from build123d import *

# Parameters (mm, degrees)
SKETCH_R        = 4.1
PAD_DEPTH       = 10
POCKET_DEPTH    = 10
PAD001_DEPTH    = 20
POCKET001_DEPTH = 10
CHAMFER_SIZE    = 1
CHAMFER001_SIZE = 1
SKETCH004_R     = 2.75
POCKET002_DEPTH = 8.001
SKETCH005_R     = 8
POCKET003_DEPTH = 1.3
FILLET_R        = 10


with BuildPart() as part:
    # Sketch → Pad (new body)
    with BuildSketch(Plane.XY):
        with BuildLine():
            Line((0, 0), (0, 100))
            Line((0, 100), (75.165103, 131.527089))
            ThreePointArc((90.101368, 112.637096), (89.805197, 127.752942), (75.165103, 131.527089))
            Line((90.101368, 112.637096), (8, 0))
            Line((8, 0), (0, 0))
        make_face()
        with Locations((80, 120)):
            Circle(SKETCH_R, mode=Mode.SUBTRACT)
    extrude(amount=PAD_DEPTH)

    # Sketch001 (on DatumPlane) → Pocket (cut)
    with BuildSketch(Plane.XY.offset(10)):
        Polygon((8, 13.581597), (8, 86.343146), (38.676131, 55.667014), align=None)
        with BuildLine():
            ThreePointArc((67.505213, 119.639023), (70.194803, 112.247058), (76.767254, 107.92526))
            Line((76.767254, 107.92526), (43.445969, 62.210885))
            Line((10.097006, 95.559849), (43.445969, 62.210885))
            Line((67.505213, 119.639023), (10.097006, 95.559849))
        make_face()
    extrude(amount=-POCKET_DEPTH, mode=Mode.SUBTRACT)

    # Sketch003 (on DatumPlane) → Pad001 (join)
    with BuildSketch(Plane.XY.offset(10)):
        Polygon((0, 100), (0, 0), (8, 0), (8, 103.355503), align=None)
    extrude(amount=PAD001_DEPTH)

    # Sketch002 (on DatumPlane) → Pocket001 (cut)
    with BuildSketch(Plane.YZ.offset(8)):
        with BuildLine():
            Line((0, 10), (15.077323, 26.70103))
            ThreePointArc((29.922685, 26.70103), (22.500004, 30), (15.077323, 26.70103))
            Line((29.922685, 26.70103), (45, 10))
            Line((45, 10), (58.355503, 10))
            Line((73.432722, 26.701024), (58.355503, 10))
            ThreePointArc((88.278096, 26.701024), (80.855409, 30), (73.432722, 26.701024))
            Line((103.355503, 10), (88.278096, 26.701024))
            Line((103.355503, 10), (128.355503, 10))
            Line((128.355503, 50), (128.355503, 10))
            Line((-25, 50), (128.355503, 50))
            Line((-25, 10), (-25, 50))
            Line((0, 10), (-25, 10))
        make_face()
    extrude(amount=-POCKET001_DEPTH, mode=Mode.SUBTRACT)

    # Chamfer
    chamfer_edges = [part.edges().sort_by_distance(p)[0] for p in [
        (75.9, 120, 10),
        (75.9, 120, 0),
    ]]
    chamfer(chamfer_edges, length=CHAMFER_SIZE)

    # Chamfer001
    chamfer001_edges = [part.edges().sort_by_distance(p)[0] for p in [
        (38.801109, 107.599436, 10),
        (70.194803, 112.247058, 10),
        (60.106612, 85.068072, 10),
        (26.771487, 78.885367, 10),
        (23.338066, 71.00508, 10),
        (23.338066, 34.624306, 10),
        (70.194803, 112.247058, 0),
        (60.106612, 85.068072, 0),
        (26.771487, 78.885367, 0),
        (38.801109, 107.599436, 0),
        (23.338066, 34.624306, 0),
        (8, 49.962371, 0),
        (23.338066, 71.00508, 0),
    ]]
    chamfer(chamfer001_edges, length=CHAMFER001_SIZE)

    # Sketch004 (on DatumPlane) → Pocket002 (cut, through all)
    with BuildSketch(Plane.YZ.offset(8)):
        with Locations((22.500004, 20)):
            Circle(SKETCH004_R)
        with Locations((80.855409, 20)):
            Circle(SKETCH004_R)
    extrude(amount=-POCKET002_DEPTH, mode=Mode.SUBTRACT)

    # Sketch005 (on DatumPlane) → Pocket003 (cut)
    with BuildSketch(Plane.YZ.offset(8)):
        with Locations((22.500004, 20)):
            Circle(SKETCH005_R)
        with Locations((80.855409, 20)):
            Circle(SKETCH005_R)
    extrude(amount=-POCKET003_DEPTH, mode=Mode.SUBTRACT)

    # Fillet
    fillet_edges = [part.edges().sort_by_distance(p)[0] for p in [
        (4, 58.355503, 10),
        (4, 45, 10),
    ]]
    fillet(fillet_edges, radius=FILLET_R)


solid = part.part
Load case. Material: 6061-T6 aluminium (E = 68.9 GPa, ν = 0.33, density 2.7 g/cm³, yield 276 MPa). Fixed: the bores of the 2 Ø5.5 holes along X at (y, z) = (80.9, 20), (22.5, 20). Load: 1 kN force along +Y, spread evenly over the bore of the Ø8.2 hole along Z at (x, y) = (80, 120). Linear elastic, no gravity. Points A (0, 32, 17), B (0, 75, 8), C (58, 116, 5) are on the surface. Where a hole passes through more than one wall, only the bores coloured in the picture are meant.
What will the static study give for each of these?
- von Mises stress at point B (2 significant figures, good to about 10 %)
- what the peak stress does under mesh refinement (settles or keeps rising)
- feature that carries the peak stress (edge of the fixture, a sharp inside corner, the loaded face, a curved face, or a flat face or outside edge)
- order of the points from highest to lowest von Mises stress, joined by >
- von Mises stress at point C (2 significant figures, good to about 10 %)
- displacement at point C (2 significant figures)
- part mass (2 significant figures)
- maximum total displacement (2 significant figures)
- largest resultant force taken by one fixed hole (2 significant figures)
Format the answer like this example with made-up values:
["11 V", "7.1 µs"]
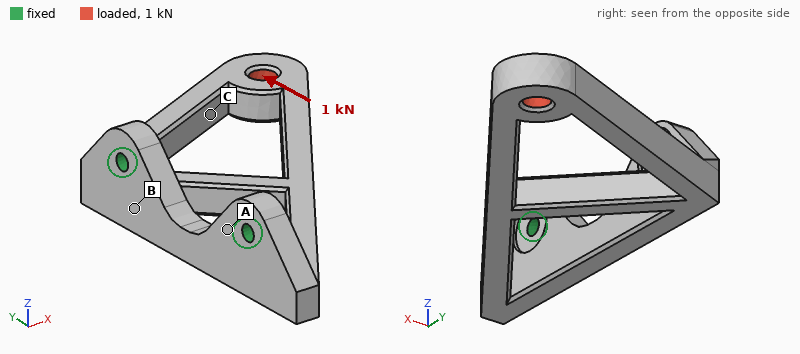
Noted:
["27 MPa", "keeps rising", "edge of the fixture", "C > B > A", "43 MPa", "0.24 mm", "110 g", "0.27 mm", "1.2 kN"]
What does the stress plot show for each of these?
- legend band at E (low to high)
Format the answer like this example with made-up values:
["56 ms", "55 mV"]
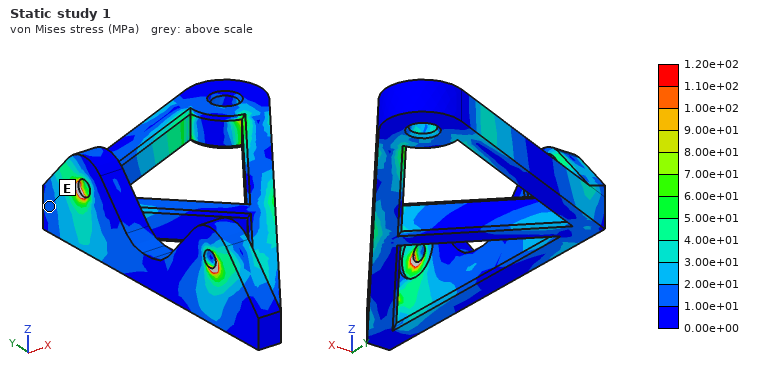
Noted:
["1.00e+01 to 2.00e+01 MPa"]
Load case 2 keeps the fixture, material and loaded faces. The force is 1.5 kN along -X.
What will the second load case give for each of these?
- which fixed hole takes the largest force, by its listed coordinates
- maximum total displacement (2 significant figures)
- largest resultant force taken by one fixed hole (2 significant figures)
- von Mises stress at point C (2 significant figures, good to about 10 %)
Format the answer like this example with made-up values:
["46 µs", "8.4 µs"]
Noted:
["(80.9, 20)", "0.48 mm", "2.1 kN", "66 MPa"]
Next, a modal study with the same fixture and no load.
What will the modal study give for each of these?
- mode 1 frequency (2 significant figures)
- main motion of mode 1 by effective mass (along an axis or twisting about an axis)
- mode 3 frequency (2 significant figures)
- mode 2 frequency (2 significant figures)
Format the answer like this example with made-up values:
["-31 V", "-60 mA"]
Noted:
["590 Hz", "along Z", "2100 Hz", "1700 Hz"]
